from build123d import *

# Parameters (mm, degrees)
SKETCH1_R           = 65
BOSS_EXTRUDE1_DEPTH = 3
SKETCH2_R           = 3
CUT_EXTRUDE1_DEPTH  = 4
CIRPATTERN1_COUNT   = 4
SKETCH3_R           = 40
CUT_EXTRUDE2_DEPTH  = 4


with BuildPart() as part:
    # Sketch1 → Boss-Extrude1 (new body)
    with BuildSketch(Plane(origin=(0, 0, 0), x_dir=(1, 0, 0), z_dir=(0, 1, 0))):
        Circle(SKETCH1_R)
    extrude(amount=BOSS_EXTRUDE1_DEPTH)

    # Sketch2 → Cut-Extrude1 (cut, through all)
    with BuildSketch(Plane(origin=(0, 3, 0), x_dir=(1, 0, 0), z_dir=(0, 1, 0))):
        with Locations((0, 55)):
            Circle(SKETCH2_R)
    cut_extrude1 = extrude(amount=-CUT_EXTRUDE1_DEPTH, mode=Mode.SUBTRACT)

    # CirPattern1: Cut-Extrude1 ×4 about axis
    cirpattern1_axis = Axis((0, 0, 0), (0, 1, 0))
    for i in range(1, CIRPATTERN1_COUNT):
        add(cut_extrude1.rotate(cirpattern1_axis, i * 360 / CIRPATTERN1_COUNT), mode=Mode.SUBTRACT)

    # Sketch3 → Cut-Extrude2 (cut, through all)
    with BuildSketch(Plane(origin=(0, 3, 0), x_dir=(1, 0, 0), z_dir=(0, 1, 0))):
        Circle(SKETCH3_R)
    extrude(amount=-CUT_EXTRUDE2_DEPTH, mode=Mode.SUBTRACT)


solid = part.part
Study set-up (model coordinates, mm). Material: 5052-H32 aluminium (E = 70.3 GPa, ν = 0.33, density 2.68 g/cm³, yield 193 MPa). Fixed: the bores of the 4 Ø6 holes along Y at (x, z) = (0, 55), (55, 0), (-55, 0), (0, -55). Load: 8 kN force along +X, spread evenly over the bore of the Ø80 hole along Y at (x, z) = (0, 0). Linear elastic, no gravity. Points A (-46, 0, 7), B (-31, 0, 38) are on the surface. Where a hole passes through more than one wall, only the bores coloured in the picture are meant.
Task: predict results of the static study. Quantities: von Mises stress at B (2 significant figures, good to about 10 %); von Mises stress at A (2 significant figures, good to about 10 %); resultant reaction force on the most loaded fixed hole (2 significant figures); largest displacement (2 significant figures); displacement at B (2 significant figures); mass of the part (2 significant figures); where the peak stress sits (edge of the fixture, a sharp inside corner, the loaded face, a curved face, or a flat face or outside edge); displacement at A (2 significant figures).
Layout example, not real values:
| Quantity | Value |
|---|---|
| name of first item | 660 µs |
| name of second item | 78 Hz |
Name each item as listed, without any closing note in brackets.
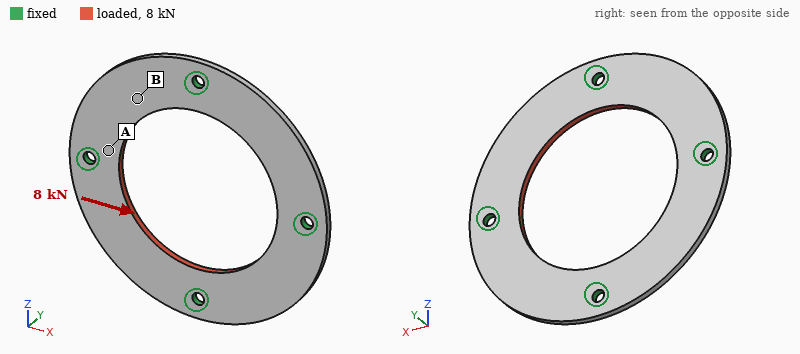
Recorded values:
| Quantity | Value |
|---|---|
| von Mises stress at B | 9.3 MPa |
| von Mises stress at A | 26 MPa |
| resultant reaction force on the most loaded fixed hole | 2.4 kN |
| largest displacement | 17 µm |
| displacement at B | 16 µm |
| mass of the part | 65 g |
| where the peak stress sits | edge of the fixture |
| displacement at A | 5.1 µm |
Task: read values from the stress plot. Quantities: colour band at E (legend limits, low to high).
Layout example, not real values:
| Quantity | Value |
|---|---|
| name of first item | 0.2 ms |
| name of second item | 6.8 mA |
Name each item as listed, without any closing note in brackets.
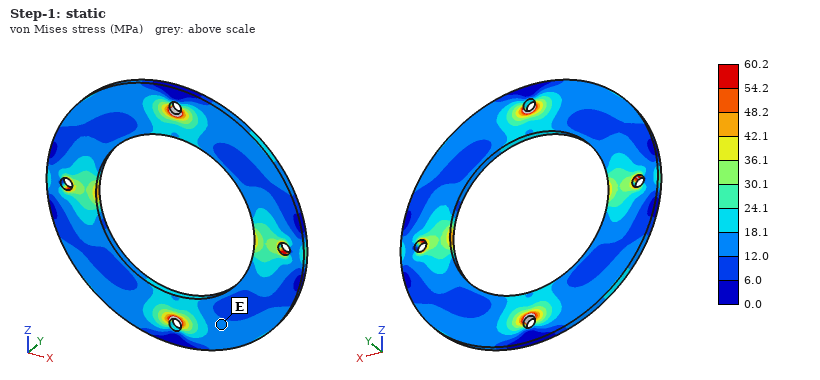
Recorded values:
| Quantity | Value |
|---|---|
| colour band at E | 12.0 to 18.1 MPa |
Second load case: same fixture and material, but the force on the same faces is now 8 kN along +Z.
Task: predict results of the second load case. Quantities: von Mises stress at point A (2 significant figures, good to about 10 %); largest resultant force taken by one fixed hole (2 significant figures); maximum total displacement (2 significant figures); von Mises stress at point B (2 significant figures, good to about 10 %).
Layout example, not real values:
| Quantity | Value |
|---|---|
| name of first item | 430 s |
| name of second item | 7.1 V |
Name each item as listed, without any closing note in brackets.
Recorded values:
| Quantity | Value |
|---|---|
| von Mises stress at point A | 23 MPa |
| largest resultant force taken by one fixed hole | 2.4 kN |
| maximum total displacement | 17 µm |
| von Mises stress at point B | 11 MPa |
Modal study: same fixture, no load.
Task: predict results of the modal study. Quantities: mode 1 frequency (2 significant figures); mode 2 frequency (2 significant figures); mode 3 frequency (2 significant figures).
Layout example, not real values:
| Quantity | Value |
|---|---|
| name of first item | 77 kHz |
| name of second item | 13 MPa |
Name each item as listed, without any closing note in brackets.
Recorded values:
| Quantity | Value |
|---|---|
| mode 1 frequency | 2100 Hz |
| mode 2 frequency | 2100 Hz |
| mode 3 frequency | 2100 Hz |
